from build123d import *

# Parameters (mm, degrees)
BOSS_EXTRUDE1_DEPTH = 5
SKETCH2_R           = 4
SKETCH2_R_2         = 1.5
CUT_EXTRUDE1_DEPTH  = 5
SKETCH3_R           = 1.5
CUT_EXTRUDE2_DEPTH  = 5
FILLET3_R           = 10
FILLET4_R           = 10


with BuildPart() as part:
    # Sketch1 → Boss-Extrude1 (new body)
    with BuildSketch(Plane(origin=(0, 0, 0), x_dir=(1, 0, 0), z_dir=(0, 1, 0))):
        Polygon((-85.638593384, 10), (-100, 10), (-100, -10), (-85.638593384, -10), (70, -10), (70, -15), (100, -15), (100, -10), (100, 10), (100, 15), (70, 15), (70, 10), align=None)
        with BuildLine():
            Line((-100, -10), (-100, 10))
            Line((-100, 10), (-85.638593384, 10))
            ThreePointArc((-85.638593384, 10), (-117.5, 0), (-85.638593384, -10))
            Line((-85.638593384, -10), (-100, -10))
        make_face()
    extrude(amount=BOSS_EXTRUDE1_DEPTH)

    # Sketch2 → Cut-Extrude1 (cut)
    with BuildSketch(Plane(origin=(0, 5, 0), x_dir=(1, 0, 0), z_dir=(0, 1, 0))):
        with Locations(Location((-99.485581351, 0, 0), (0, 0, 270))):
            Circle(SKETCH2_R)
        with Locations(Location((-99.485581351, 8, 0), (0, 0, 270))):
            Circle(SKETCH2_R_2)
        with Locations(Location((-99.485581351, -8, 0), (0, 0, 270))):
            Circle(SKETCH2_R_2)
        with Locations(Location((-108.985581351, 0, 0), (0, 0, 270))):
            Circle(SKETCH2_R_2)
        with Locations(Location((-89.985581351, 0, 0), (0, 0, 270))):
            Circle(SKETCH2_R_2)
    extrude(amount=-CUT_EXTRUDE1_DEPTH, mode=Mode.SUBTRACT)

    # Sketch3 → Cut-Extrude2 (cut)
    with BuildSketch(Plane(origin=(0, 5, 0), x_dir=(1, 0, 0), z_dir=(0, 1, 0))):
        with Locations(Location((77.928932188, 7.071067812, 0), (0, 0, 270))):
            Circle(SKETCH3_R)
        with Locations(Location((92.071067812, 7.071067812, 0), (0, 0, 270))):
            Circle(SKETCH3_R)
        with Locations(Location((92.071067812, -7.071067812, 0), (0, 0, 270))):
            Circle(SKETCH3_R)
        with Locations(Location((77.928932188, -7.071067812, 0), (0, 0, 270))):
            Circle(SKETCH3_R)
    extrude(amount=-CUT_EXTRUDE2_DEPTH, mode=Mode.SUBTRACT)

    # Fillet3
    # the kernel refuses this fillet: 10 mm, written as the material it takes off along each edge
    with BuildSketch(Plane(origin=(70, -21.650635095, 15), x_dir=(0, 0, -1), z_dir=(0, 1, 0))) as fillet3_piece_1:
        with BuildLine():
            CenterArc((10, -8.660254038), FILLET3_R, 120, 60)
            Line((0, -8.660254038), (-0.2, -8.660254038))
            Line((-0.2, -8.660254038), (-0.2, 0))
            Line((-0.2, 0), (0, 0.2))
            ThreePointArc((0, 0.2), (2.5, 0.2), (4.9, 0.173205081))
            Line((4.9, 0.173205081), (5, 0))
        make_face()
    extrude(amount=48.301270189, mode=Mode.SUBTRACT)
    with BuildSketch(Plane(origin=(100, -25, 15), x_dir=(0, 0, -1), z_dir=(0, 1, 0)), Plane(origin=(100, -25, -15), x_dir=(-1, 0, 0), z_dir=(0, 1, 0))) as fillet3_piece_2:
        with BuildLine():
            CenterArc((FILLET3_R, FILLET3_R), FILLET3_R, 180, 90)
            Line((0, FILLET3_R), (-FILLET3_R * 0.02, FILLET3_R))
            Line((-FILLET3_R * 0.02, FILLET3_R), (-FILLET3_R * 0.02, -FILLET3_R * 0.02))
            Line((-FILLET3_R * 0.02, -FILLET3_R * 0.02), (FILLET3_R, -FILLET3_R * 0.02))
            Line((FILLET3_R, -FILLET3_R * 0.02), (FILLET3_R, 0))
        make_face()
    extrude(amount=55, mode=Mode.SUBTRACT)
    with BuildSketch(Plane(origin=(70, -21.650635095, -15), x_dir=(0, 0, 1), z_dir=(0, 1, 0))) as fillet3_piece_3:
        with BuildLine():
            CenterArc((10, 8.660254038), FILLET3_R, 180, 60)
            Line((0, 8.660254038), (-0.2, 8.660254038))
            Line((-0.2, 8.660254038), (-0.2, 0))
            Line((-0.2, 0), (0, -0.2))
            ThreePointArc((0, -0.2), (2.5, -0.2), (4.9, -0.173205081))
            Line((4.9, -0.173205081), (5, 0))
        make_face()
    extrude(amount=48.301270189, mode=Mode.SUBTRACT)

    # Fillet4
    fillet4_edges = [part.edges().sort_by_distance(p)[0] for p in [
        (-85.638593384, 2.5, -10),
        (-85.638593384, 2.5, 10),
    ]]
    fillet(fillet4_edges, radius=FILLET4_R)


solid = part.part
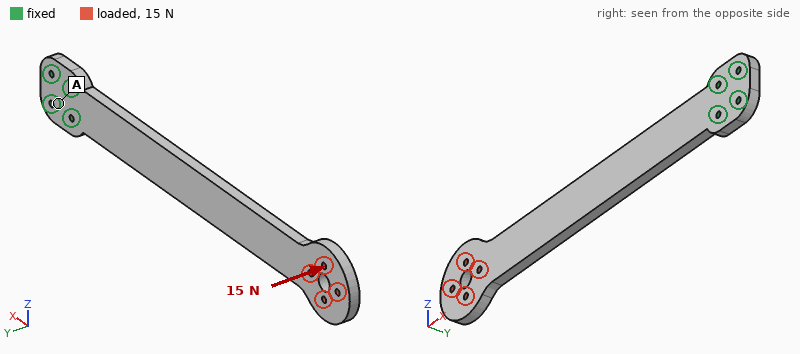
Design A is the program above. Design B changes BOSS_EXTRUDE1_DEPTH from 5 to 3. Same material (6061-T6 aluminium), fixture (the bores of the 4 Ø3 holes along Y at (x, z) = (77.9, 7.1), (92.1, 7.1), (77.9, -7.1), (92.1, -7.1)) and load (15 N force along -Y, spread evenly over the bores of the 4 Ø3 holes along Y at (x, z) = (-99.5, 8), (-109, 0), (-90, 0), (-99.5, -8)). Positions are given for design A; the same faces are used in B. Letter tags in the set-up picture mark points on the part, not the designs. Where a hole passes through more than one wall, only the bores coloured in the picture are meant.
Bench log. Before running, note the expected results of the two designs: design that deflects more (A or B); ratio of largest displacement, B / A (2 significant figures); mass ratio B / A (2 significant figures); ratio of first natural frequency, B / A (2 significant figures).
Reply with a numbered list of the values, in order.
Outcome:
1. B
2. 4.6
3. 0.60
4. 0.60
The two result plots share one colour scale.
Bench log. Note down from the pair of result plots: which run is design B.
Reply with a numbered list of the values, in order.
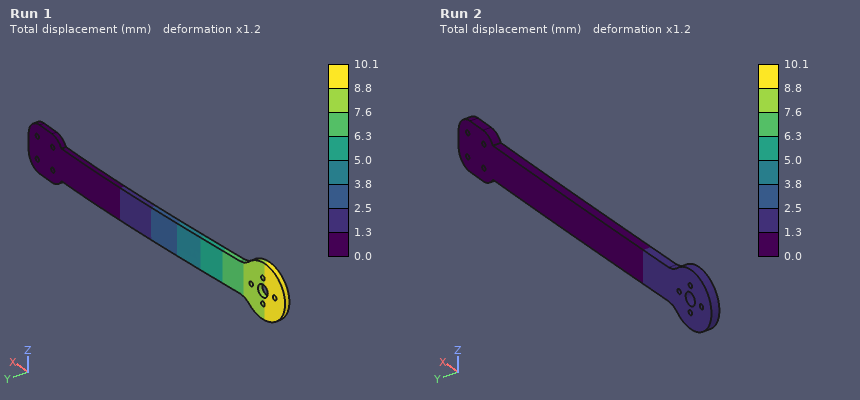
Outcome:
1. Run 1
